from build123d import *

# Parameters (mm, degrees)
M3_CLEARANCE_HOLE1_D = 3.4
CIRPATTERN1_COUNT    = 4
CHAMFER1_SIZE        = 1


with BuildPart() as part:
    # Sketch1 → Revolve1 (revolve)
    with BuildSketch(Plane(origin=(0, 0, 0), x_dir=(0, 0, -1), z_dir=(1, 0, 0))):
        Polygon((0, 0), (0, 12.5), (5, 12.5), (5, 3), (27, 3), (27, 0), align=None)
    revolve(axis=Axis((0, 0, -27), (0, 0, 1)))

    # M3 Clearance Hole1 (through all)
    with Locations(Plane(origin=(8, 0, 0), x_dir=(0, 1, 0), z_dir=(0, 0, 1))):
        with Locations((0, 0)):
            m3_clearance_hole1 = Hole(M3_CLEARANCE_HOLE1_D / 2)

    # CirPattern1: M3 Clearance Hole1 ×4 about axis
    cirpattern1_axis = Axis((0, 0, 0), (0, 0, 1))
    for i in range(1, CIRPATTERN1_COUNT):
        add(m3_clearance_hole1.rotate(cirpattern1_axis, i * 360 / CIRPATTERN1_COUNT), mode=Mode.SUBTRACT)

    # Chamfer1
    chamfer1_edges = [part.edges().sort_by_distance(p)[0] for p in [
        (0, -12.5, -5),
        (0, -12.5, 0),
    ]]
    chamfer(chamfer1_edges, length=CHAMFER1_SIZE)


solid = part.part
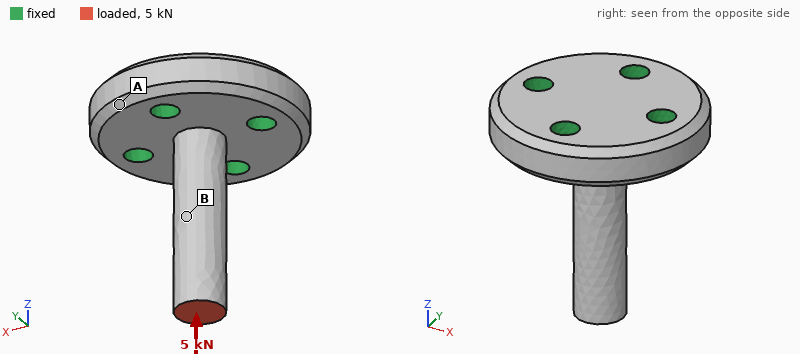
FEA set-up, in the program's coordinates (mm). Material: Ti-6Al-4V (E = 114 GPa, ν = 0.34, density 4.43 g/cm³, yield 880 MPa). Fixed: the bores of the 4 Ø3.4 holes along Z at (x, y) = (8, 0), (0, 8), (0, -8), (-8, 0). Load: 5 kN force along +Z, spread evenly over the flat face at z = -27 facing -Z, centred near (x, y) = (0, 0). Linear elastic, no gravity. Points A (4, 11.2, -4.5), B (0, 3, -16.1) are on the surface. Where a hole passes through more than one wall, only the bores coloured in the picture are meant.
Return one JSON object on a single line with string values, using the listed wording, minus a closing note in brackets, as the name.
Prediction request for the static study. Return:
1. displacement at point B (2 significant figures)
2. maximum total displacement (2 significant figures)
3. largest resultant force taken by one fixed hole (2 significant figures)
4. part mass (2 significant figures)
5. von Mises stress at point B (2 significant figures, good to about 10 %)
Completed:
{"displacement at point B": "25 µm", "maximum total displacement": "42 µm", "largest resultant force taken by one fixed hole": "1.3 kN", "part mass": "12 g", "von Mises stress at point B": "180 MPa"}
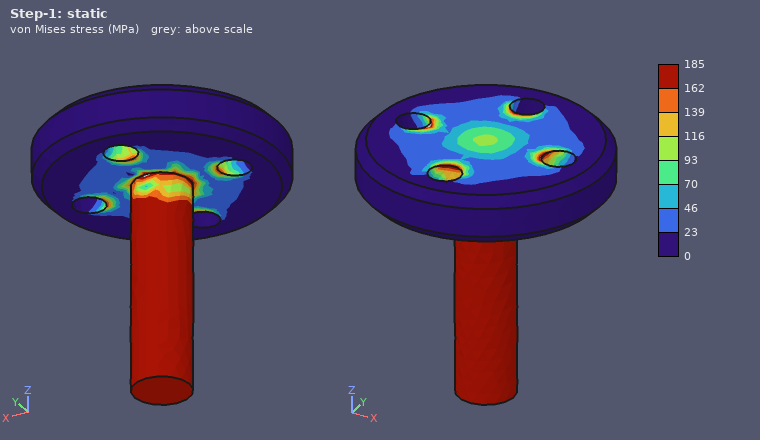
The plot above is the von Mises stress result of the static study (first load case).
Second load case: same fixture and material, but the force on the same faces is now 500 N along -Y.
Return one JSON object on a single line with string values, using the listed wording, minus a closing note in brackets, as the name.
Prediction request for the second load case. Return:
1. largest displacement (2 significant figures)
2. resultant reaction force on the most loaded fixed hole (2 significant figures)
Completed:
{"largest displacement": "0.31 mm", "resultant reaction force on the most loaded fixed hole": "890 N"}
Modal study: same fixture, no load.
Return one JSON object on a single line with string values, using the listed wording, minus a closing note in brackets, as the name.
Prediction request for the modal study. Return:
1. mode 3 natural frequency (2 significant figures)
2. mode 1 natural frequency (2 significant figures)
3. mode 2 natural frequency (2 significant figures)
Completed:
{"mode 3 natural frequency": "34 kHz", "mode 1 natural frequency": "7500 Hz", "mode 2 natural frequency": "7500 Hz"}
